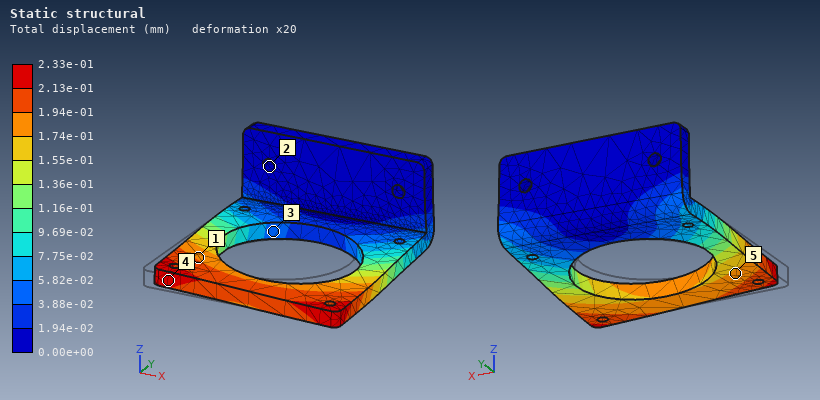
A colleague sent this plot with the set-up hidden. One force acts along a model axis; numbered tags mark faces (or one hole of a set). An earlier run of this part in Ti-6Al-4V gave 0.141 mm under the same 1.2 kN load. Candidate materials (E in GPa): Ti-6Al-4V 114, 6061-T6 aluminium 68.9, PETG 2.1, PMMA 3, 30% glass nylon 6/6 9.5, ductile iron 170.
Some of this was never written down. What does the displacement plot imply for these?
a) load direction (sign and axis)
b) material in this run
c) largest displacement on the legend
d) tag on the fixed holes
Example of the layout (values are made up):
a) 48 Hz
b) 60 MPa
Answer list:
a) +X
b) 6061-T6 aluminium
c) 2.33e-01 mm
d) 2
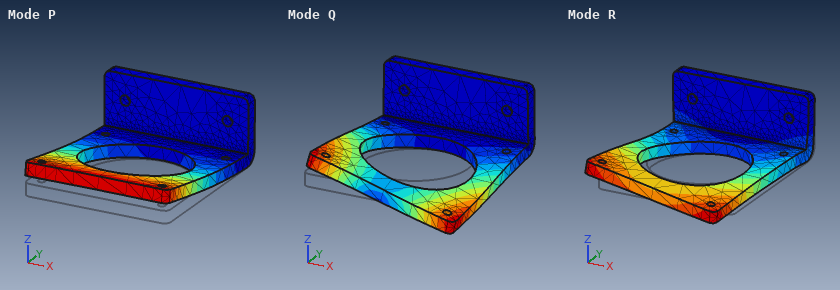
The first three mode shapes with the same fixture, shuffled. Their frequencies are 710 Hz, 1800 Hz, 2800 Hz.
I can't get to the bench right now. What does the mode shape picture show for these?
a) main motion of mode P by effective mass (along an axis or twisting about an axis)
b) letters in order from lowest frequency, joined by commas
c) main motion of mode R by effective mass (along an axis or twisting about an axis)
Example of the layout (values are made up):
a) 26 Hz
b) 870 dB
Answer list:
a) along Z
b) P, Q, R
c) along X
